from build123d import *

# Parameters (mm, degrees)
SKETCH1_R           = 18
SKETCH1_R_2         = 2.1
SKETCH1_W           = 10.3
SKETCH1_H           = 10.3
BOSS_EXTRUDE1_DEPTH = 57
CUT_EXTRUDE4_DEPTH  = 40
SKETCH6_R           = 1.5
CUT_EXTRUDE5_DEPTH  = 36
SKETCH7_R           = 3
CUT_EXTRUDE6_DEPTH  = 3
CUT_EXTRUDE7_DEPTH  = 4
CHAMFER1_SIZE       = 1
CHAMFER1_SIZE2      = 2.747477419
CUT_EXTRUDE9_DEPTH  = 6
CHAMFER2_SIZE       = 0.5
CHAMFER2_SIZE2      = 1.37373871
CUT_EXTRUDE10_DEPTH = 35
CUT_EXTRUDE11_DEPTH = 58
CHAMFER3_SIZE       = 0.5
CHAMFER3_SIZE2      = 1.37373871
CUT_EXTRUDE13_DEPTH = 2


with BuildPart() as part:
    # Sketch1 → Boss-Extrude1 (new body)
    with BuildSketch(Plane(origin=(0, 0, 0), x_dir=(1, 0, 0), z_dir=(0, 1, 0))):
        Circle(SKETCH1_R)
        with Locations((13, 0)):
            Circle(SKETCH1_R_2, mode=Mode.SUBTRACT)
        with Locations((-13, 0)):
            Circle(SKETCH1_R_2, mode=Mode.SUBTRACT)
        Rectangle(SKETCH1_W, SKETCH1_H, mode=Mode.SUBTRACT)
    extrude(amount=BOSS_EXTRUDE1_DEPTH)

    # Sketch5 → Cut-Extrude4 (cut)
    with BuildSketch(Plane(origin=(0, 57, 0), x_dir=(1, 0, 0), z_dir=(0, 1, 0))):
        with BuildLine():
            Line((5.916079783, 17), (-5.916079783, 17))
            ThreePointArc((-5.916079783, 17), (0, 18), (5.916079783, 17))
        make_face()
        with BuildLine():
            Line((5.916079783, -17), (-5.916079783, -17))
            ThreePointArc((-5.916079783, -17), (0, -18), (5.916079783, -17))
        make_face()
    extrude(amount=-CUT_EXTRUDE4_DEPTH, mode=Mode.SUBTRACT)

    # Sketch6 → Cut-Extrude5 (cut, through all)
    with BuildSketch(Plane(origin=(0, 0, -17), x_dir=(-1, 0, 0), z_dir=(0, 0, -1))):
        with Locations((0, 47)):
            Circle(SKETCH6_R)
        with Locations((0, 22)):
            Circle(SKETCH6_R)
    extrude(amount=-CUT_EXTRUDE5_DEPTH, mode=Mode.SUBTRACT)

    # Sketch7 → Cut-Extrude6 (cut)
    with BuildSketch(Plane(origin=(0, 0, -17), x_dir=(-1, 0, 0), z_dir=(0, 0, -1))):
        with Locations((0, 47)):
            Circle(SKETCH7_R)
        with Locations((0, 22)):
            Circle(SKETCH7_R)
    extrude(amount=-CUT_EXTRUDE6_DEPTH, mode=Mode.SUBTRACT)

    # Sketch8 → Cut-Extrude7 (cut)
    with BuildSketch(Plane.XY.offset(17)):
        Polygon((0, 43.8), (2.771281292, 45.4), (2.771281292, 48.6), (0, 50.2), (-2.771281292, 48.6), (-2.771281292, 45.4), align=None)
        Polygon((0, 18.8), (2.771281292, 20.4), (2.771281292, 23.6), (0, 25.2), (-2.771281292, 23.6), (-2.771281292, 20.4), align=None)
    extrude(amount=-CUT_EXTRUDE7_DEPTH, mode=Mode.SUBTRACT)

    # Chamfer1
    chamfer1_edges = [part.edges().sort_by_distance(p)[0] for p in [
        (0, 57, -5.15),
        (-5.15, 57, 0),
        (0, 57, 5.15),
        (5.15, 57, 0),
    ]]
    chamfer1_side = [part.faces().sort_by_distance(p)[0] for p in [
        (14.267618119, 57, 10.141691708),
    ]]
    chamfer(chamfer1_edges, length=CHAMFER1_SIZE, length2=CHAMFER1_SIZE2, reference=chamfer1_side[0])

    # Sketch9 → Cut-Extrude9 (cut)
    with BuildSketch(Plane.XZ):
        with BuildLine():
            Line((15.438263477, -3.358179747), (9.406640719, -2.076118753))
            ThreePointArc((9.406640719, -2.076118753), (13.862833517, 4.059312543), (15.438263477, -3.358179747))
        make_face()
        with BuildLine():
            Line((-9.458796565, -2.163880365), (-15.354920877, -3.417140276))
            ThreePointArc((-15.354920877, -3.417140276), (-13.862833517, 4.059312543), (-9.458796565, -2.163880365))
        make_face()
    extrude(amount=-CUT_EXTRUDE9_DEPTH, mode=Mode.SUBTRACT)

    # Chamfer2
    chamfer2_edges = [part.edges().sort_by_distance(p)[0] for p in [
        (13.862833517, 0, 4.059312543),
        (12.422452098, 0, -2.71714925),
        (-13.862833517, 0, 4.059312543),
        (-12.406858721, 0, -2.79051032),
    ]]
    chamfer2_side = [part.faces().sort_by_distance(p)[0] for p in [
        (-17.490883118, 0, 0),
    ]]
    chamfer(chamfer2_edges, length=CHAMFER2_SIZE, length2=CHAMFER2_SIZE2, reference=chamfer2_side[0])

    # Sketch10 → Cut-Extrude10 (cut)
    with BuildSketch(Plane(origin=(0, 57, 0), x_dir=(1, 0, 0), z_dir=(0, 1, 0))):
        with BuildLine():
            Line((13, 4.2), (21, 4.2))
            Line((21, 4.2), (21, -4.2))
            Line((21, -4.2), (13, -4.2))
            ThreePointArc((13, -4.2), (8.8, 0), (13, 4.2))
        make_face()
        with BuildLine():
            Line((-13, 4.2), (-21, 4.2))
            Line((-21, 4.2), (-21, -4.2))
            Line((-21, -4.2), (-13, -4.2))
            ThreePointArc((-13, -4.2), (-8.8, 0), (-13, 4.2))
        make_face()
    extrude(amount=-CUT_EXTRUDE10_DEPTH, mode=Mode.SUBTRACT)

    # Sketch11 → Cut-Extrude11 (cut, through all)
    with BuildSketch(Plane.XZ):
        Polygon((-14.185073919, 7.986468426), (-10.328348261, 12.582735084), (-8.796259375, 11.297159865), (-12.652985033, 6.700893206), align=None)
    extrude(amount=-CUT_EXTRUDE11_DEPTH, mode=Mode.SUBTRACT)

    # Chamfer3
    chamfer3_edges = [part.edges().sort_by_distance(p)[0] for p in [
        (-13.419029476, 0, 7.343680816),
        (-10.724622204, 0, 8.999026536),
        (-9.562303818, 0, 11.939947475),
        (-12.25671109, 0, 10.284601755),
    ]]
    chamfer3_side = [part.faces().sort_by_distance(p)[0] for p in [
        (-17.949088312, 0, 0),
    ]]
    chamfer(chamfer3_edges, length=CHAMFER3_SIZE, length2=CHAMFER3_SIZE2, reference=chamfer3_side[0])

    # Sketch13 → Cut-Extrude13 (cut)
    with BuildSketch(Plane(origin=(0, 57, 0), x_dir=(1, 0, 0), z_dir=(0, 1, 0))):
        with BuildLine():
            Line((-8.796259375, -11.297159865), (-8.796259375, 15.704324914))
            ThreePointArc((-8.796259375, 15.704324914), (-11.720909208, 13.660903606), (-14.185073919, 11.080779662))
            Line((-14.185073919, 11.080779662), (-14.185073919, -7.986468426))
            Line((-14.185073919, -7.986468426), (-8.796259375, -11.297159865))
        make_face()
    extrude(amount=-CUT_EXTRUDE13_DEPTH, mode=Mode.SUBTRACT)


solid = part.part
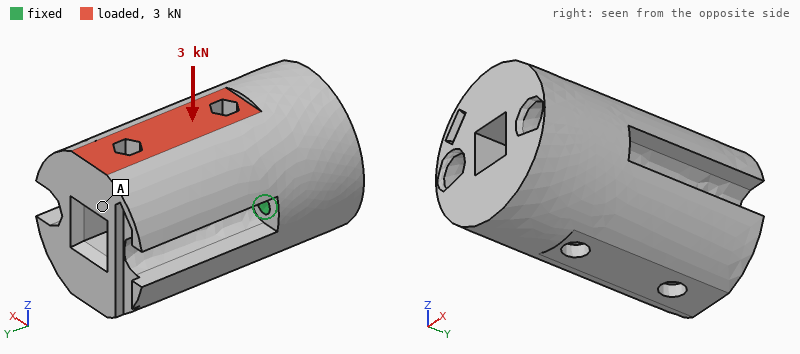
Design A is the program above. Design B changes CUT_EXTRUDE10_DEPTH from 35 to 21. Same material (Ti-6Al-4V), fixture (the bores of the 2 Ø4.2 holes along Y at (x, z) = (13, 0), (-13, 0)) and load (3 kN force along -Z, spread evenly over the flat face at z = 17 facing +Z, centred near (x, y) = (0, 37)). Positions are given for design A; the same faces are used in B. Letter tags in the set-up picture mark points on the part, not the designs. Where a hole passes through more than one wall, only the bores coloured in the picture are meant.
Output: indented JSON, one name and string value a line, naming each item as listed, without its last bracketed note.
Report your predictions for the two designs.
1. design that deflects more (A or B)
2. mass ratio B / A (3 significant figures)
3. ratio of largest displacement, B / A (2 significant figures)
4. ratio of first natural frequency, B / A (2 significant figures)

{
  "design that deflects more": "A",
  "mass ratio B / A": "1.03",
  "ratio of largest displacement, B / A": "0.27",
  "ratio of first natural frequency, B / A": "2.2"
}
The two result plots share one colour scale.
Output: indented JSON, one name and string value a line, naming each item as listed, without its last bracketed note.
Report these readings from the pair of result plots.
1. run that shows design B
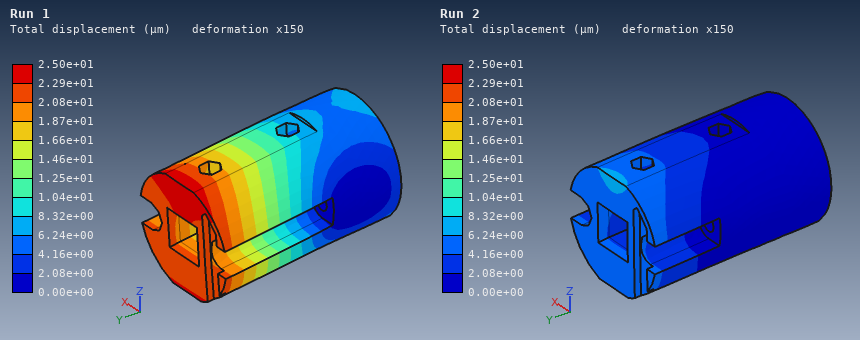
{
  "run that shows design B": "Run 2"
}
